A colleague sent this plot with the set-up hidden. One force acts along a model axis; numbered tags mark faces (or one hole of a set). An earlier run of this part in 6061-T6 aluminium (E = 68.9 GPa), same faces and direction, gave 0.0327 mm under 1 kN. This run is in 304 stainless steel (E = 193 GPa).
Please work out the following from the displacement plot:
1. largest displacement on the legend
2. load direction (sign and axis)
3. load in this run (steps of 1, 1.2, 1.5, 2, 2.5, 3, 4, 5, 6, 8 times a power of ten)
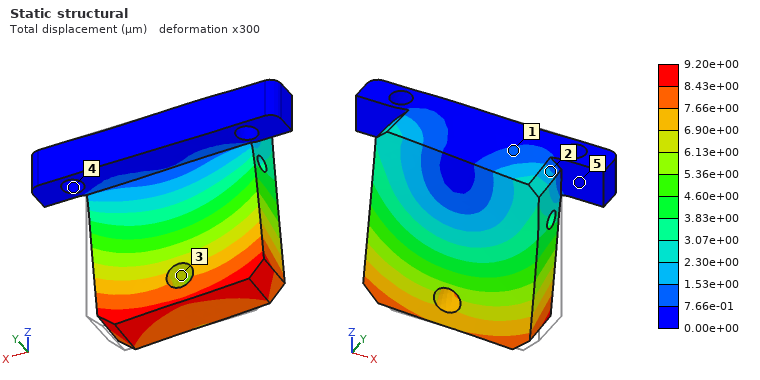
9.20e+00 µm
-X
800 N
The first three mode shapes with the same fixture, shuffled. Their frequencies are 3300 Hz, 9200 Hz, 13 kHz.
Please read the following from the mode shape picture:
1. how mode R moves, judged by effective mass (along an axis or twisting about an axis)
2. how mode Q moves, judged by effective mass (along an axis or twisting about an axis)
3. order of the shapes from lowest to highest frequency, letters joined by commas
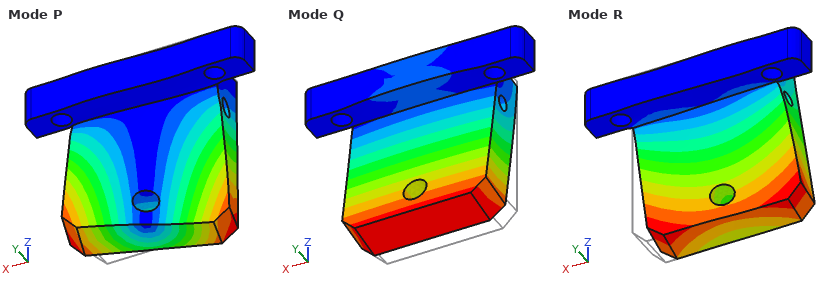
along X
along Y
Q, R, P
